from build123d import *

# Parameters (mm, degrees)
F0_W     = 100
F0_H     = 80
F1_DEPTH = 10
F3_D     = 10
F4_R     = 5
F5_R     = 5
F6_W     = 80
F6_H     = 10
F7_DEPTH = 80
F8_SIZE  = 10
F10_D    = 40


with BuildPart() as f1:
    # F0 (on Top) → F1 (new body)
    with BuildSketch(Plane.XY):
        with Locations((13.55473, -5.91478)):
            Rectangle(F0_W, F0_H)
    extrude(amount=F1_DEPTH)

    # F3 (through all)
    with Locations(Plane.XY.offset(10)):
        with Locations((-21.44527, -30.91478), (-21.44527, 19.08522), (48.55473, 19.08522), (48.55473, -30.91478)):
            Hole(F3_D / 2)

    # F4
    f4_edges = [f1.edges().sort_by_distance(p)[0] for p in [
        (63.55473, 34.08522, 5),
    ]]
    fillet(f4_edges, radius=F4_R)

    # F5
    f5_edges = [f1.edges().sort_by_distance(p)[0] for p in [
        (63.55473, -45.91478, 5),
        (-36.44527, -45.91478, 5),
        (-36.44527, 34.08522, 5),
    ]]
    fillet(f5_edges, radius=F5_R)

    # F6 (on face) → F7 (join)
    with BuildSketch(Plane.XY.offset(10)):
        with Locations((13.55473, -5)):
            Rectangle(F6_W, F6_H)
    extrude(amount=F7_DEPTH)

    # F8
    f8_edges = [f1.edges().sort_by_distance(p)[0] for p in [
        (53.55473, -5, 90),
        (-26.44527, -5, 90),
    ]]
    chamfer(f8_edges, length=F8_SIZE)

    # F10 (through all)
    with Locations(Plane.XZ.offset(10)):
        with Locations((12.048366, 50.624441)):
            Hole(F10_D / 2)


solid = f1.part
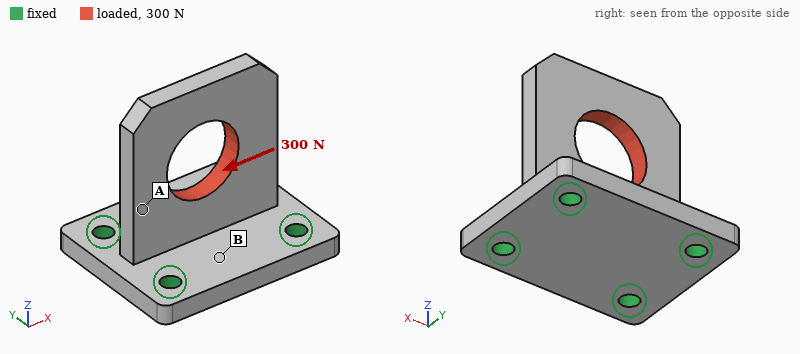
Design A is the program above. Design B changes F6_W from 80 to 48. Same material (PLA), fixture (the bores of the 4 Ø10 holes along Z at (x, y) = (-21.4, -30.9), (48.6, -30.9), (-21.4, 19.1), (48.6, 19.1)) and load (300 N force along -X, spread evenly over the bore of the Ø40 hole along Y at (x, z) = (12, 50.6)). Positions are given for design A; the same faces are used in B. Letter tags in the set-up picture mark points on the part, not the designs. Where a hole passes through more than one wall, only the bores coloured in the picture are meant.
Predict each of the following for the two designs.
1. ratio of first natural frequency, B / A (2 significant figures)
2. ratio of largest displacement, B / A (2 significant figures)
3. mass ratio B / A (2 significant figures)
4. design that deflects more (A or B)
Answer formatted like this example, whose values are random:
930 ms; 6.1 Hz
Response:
0.87; 5.8; 0.80; B
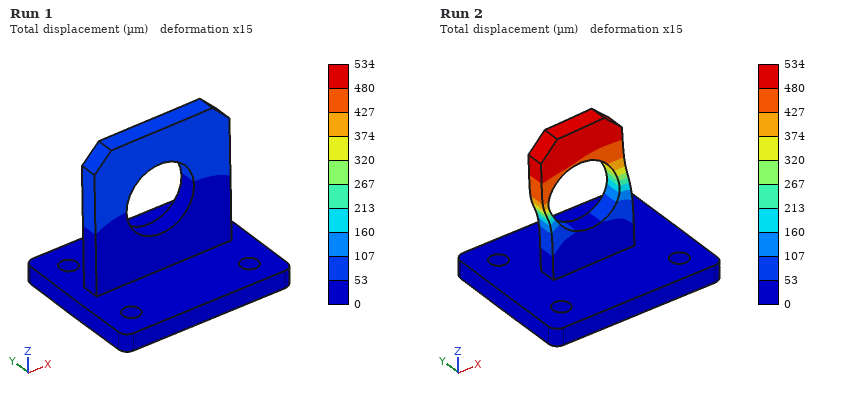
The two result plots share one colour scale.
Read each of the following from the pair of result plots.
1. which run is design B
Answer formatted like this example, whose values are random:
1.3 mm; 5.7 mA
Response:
Run 2
